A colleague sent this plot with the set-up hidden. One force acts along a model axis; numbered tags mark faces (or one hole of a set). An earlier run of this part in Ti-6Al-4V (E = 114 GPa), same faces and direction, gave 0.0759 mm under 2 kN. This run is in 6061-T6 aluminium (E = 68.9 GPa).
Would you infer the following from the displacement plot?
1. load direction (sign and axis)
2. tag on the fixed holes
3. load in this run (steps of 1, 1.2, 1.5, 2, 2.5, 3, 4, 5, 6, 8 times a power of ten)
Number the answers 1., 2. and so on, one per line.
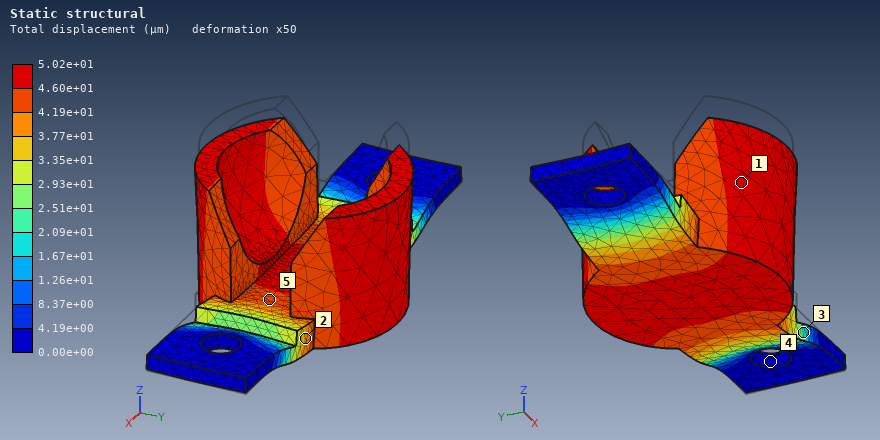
1. -Z
2. 4
3. 800 N
